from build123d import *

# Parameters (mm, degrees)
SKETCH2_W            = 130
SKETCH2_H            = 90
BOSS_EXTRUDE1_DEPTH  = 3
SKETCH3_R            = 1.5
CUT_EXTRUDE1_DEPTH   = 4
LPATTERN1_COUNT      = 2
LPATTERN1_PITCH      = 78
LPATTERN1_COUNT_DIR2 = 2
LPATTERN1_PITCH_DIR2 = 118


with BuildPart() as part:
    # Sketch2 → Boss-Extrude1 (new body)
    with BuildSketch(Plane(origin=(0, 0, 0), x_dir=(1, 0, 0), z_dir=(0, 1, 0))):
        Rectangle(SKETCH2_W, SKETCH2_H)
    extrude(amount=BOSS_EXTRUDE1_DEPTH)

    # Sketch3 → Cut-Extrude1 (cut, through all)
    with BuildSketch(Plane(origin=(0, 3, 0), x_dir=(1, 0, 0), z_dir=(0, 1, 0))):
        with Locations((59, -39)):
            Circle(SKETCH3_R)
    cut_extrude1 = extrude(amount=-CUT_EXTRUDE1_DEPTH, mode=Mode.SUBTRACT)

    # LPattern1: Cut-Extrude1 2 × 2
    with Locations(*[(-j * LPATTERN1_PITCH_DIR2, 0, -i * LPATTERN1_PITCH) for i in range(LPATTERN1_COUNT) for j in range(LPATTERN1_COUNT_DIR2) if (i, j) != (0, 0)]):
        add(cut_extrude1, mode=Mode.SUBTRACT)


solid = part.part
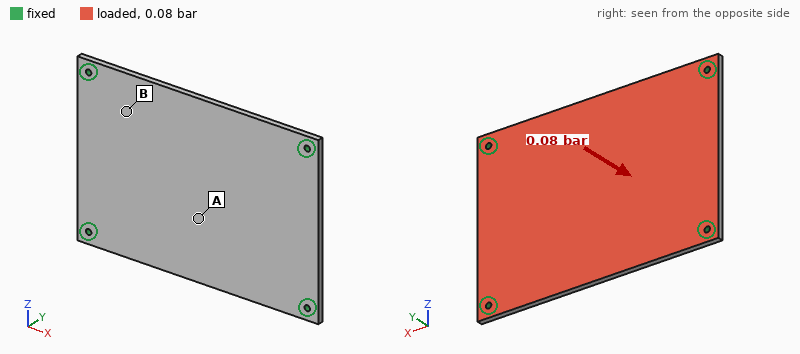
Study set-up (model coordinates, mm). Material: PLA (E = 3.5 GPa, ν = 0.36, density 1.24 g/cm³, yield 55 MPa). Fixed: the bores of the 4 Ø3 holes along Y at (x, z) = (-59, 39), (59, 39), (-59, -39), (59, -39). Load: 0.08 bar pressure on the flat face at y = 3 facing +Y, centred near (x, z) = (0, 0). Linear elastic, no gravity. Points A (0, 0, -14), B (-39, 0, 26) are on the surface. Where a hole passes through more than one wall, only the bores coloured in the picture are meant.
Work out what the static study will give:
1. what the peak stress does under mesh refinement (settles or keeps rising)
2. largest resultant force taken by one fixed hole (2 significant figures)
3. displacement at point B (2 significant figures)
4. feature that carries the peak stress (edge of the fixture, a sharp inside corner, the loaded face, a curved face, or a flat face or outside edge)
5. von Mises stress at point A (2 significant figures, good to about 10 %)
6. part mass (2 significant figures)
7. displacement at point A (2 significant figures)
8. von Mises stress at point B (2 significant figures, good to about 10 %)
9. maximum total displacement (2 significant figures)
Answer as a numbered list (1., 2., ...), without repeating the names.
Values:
1. keeps rising
2. 23 N
3. 0.38 mm
4. edge of the fixture
5. 3.6 MPa
6. 43 g
7. 0.86 mm
8. 1.1 MPa
9. 0.87 mm
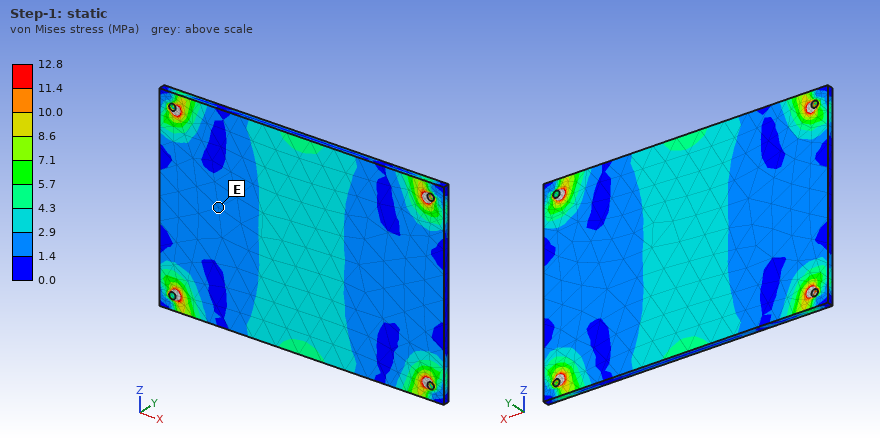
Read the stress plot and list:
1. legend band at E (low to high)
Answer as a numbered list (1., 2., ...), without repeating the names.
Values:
1. 1.4 to 2.9 MPa
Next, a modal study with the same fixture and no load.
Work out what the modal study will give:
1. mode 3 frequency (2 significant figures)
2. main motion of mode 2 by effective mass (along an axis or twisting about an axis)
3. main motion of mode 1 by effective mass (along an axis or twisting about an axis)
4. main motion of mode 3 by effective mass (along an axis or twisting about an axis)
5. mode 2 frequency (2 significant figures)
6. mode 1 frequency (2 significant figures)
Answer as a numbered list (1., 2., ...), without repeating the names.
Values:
1. 710 Hz
2. twisting about X
3. along Y
4. twisting about Z
5. 480 Hz
6. 290 Hz
